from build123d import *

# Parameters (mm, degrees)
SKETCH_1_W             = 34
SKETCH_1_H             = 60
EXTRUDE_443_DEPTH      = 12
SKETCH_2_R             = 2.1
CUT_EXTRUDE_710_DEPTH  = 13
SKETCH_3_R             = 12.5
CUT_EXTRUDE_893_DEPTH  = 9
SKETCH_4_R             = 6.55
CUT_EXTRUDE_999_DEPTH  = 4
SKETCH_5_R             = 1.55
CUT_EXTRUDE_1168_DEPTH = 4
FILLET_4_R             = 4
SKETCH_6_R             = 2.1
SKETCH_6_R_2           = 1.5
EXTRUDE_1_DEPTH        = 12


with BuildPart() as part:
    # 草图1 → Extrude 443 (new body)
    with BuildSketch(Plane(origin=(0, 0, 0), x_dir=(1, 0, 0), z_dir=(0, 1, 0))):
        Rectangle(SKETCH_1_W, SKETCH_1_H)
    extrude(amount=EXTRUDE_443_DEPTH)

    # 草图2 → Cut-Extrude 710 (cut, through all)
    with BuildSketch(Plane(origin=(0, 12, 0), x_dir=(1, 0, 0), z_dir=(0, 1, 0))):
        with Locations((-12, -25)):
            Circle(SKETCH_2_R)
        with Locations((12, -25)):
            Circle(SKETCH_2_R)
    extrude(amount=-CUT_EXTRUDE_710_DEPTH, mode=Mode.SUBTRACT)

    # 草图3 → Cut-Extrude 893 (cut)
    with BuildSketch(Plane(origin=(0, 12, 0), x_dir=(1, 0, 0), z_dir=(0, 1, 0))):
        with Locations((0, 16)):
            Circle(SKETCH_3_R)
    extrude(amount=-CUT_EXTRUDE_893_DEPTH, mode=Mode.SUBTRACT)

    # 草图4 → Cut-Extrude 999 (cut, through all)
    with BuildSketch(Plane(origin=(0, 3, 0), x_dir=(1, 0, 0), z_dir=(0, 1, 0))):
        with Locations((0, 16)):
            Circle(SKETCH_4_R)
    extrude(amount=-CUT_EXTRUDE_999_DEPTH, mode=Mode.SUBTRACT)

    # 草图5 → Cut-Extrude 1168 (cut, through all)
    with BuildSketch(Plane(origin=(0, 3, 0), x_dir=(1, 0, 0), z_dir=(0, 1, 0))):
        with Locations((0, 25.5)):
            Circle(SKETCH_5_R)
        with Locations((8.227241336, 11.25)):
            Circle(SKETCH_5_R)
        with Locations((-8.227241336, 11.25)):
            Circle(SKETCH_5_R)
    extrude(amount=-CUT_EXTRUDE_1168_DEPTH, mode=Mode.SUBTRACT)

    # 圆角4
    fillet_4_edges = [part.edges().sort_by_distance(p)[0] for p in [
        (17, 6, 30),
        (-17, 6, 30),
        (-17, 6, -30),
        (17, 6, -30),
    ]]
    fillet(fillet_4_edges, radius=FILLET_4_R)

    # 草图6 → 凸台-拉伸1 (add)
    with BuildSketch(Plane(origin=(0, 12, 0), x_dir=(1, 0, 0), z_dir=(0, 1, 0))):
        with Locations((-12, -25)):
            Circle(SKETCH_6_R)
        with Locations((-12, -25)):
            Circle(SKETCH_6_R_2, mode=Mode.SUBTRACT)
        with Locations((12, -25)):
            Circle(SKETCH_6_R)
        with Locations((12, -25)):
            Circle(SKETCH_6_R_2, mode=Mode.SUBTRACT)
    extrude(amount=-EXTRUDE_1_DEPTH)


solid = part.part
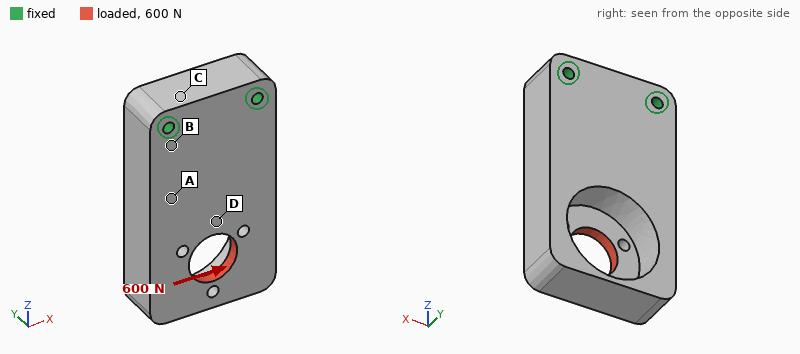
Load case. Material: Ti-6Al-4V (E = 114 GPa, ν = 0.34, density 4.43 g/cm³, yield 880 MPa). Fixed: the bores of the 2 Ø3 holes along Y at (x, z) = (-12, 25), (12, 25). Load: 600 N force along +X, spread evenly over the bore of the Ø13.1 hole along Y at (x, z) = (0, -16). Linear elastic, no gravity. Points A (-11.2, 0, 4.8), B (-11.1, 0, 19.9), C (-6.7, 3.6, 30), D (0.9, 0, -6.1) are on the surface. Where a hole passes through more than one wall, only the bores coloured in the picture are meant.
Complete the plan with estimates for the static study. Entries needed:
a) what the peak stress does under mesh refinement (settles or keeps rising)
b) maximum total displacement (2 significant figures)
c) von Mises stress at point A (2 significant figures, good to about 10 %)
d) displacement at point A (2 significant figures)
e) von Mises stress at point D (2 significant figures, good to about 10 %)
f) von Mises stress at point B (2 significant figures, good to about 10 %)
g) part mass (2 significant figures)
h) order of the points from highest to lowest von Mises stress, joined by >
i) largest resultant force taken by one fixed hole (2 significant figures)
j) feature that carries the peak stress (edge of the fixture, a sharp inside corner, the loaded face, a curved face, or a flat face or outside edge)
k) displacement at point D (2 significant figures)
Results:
keeps rising
11 µm
5.4 MPa
2.5 µm
14 MPa
7.5 MPa
85 g
D > B > A > C
1.0 kN
edge of the fixture
4.3 µm
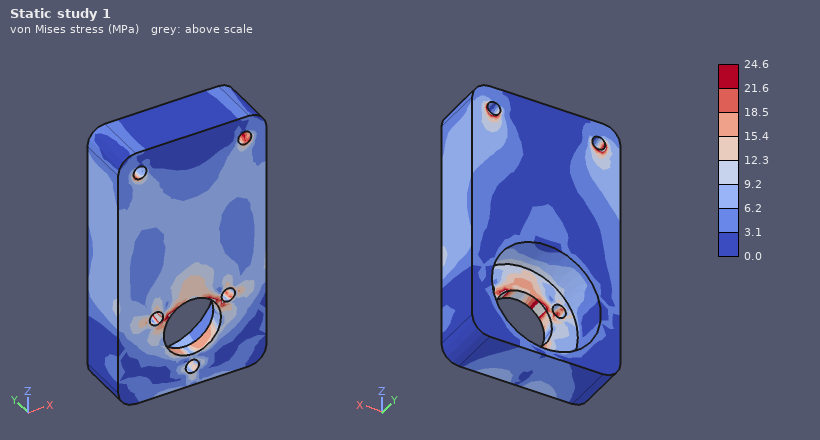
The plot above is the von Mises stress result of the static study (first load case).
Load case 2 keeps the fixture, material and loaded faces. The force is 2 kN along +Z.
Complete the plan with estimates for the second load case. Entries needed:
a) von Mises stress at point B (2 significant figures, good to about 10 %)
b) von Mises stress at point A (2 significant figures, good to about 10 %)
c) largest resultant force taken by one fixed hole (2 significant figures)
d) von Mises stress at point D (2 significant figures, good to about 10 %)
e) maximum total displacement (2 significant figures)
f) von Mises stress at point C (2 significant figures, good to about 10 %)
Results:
24 MPa
17 MPa
1.0 kN
20 MPa
28 µm
6.7 MPa
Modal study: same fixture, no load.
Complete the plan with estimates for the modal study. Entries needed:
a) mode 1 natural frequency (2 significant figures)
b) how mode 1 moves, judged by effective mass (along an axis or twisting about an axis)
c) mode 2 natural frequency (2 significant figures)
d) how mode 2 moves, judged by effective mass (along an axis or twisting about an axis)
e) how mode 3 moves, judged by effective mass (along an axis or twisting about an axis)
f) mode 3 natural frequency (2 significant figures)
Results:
3500 Hz
along Y
7100 Hz
along X
along X
8500 Hz
